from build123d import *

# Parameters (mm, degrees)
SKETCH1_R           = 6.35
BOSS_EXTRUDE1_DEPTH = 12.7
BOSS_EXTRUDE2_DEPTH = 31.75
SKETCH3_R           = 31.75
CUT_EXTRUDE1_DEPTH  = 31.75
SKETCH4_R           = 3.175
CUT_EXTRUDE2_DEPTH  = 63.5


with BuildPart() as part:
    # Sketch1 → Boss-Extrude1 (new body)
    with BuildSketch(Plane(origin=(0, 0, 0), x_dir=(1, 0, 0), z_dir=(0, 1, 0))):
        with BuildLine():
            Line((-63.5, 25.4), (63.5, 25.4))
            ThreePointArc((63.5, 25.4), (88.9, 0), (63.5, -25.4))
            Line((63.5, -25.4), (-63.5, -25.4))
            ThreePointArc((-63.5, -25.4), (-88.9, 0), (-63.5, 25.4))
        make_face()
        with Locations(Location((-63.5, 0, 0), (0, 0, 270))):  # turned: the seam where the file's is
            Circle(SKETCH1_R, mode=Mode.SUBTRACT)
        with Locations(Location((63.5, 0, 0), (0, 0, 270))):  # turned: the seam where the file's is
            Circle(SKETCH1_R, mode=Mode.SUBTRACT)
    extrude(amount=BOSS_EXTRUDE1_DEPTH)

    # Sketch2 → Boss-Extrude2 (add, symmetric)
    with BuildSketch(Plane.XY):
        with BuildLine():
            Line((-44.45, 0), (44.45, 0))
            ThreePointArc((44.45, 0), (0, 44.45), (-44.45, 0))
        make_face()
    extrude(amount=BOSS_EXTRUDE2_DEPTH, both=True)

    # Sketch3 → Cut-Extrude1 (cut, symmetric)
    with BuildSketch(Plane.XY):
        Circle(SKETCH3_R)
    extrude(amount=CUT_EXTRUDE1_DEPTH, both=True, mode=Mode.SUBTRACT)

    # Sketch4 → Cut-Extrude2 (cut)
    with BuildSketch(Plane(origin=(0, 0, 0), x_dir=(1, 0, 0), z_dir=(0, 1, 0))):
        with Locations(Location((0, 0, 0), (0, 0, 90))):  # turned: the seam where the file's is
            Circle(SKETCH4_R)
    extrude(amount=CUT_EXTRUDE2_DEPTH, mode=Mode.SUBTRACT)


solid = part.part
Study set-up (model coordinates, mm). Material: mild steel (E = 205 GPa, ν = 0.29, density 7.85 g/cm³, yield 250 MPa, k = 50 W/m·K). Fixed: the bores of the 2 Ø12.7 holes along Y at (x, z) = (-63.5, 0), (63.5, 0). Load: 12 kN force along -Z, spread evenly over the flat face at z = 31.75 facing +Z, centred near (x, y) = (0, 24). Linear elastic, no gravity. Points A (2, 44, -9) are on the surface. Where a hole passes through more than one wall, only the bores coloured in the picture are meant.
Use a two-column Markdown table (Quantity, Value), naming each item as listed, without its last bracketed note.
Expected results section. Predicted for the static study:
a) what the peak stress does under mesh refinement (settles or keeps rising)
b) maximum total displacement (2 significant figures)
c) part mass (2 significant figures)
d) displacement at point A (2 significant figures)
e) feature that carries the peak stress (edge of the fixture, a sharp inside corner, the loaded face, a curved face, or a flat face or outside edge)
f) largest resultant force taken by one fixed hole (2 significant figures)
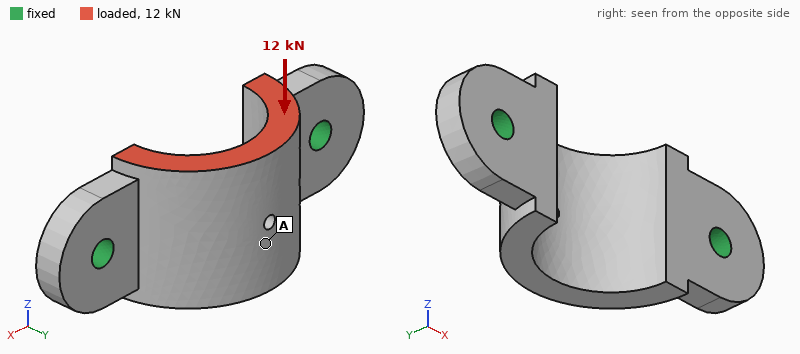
| Quantity | Value |
|---|---|
| what the peak stress does under mesh refinement | keeps rising |
| maximum total displacement | 67 µm |
| part mass | 1.1 kg |
| displacement at point A | 55 µm |
| feature that carries the peak stress | edge of the fixture |
| largest resultant force taken by one fixed hole | 6.0 kN |
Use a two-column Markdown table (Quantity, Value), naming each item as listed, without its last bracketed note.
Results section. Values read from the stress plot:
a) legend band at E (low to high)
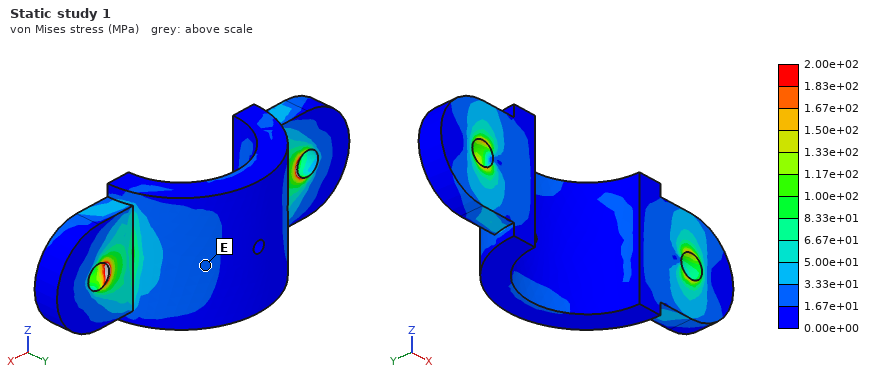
| Quantity | Value |
|---|---|
| legend band at E | 1.67e+01 to 3.33e+01 MPa |
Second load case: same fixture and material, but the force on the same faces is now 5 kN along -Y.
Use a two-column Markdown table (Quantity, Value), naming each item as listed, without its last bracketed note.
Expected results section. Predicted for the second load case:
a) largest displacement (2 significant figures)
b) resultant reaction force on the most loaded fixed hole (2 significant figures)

| Quantity | Value |
|---|---|
| largest displacement | 40 µm |
| resultant reaction force on the most loaded fixed hole | 3.2 kN |
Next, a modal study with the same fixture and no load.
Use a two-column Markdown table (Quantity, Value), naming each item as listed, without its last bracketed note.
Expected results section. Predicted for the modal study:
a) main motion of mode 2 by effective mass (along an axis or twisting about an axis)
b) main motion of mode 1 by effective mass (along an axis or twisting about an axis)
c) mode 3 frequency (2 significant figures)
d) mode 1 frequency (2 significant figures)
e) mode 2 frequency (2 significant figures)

| Quantity | Value |
|---|---|
| main motion of mode 2 by effective mass | along Y |
| main motion of mode 1 by effective mass | along Z |
| mode 3 frequency | 6900 Hz |
| mode 1 frequency | 2800 Hz |
| mode 2 frequency | 5800 Hz |
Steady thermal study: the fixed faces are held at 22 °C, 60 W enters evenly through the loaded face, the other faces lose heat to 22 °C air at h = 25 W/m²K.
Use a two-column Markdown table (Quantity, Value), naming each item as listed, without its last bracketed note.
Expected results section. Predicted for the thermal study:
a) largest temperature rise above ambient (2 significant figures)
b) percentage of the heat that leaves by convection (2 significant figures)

| Quantity | Value |
|---|---|
| largest temperature rise above ambient | 49 K |
| percentage of the heat that leaves by convection | 21 % |
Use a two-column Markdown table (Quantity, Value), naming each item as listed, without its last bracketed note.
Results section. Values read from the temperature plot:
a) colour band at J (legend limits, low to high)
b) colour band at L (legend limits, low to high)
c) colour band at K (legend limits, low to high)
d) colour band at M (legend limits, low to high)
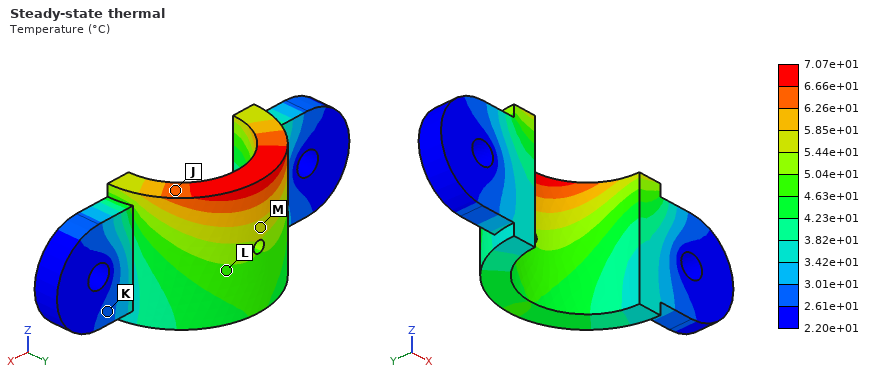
| Quantity | Value |
|---|---|
| colour band at J | 6.26e+01 to 6.66e+01 °C |
| colour band at L | 4.63e+01 to 5.04e+01 °C |
| colour band at K | 2.61e+01 to 3.01e+01 °C |
| colour band at M | 5.44e+01 to 5.85e+01 °C |
